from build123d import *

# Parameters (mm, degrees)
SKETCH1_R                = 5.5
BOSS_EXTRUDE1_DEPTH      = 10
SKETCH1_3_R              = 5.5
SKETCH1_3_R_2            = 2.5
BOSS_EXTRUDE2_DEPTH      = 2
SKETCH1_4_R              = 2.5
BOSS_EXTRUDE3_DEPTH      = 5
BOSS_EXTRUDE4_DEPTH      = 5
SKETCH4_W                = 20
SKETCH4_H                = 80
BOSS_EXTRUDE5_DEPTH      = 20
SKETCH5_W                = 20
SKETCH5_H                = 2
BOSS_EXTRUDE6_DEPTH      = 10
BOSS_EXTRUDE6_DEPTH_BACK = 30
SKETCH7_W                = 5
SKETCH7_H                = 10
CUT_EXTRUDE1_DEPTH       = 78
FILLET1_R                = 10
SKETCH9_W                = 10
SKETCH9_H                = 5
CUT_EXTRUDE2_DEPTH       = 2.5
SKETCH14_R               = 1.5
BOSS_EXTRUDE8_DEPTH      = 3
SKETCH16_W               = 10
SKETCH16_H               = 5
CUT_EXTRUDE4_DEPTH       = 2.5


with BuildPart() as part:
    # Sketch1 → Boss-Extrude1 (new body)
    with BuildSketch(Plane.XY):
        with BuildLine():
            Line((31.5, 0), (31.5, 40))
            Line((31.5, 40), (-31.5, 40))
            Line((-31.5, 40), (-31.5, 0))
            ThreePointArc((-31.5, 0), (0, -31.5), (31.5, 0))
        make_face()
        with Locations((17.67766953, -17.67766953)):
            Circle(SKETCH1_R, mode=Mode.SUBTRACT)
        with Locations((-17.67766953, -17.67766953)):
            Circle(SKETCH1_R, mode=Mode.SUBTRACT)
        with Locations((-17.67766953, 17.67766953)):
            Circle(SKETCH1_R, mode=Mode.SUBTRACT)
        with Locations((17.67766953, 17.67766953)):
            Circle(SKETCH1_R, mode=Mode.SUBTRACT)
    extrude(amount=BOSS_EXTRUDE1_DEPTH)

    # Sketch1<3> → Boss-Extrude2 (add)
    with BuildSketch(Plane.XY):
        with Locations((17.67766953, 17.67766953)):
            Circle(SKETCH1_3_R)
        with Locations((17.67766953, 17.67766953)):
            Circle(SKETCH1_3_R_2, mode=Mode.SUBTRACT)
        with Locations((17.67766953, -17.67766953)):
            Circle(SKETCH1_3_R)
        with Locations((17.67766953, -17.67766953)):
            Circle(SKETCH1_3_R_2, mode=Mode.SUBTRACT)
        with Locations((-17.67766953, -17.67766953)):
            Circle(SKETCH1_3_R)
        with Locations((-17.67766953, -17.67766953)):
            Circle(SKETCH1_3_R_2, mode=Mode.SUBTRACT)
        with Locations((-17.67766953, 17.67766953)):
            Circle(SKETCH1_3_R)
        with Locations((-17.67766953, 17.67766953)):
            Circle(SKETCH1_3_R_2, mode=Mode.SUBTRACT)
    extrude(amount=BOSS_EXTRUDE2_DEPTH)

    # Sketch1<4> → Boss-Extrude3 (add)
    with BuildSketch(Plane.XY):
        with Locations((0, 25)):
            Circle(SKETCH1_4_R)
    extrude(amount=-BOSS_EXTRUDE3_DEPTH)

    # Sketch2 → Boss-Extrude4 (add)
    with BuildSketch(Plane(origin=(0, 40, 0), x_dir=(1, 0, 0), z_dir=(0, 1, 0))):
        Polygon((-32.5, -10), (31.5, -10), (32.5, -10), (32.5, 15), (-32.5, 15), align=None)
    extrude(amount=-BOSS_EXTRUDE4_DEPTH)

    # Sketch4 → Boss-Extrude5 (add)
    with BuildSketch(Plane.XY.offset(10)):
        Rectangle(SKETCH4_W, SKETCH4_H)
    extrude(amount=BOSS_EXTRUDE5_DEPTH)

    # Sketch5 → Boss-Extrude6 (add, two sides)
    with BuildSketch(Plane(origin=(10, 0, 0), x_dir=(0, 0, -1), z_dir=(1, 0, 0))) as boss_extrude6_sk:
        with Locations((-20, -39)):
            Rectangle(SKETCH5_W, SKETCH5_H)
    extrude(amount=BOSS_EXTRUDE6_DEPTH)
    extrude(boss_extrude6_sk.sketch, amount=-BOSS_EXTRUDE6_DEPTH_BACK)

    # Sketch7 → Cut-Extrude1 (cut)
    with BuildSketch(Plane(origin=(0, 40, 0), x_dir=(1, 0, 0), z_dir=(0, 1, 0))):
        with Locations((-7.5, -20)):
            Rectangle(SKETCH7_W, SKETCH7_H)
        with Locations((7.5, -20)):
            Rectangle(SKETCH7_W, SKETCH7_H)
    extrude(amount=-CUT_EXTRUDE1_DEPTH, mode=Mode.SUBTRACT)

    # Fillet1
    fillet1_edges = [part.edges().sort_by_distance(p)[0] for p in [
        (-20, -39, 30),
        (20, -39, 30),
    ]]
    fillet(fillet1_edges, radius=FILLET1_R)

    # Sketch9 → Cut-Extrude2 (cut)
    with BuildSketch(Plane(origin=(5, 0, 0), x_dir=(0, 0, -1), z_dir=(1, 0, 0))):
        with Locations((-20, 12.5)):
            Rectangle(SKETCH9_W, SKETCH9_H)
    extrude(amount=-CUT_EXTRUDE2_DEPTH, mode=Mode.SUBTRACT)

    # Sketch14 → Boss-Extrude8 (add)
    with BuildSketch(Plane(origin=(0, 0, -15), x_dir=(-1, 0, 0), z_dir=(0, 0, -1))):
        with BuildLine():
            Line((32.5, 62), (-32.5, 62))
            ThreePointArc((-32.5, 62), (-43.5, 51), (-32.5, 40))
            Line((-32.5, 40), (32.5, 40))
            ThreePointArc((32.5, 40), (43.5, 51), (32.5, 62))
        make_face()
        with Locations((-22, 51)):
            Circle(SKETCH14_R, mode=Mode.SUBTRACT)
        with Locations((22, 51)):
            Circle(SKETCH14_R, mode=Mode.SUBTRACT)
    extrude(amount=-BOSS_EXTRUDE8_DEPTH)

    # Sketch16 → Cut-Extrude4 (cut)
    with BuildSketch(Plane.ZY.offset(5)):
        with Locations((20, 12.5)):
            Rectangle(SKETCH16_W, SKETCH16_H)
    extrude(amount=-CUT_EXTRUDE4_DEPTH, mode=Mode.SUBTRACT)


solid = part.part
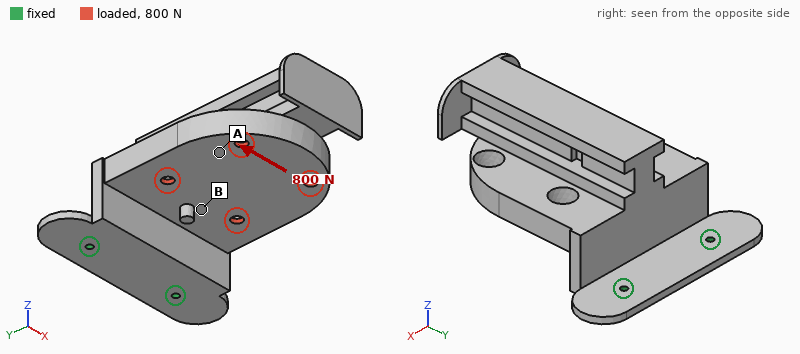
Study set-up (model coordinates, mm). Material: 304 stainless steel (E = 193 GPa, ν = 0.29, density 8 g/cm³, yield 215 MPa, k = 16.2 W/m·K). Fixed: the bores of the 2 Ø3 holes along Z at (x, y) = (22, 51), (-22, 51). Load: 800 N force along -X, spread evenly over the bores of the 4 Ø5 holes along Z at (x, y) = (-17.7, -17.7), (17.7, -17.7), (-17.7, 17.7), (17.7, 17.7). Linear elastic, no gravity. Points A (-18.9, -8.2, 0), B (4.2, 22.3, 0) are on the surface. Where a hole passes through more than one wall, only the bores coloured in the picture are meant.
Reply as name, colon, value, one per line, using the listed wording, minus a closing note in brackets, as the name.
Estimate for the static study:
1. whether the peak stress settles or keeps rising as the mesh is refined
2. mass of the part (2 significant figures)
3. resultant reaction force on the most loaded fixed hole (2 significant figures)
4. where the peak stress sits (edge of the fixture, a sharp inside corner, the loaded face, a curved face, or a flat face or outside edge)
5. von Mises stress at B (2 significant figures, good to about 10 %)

whether the peak stress settles or keeps rising as the mesh is refined: keeps rising
mass of the part: 580 g
resultant reaction force on the most loaded fixed hole: 1.0 kN
where the peak stress sits: edge of the fixture
von Mises stress at B: 10 MPa
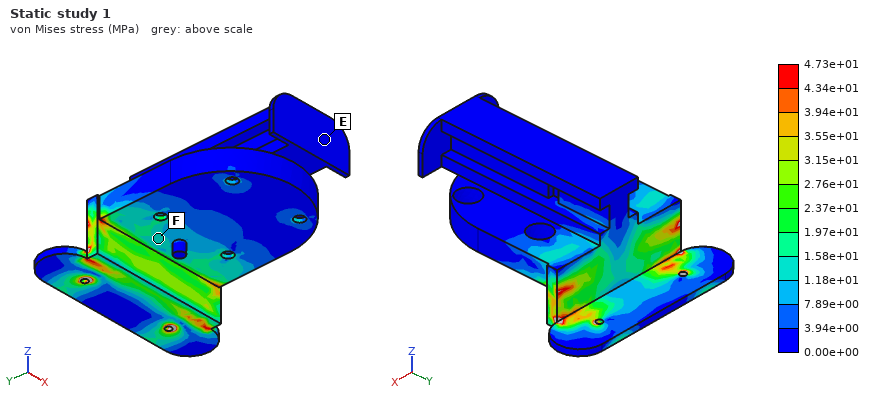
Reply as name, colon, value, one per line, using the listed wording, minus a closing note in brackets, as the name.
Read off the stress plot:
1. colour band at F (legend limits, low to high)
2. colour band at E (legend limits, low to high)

colour band at F: 1.18e+01 to 1.58e+01 MPa
colour band at E: 0.00e+00 to 3.94e+00 MPa
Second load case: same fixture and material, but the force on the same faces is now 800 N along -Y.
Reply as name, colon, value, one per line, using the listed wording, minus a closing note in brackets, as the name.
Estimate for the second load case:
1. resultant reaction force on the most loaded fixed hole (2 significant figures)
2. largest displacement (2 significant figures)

resultant reaction force on the most loaded fixed hole: 400 N
largest displacement: 0.59 mm
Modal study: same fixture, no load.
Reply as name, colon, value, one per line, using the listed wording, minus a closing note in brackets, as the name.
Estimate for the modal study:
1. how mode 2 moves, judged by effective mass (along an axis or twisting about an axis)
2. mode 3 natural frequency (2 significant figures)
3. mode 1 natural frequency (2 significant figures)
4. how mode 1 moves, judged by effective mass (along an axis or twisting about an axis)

how mode 2 moves, judged by effective mass: along X
mode 3 natural frequency: 1700 Hz
mode 1 natural frequency: 180 Hz
how mode 1 moves, judged by effective mass: along Z
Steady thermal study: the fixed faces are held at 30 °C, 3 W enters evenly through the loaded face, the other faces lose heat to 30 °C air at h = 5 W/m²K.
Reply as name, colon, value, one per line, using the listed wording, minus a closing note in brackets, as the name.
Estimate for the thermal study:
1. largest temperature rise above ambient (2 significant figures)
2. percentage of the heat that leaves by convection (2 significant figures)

largest temperature rise above ambient: 23 K
percentage of the heat that leaves by convection: 54 %
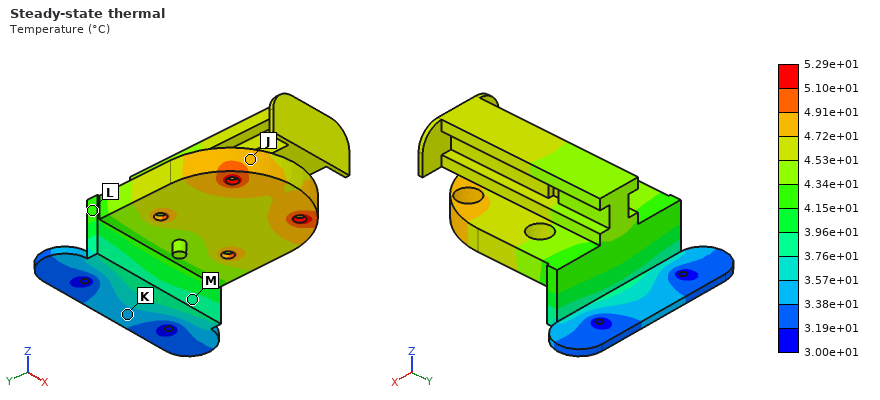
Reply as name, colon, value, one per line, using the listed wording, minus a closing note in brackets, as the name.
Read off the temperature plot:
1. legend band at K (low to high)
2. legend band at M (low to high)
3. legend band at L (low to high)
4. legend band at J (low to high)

legend band at K: 3.38e+01 to 3.57e+01 °C
legend band at M: 3.76e+01 to 3.96e+01 °C
legend band at L: 4.15e+01 to 4.34e+01 °C
legend band at J: 4.72e+01 to 4.91e+01 °C
